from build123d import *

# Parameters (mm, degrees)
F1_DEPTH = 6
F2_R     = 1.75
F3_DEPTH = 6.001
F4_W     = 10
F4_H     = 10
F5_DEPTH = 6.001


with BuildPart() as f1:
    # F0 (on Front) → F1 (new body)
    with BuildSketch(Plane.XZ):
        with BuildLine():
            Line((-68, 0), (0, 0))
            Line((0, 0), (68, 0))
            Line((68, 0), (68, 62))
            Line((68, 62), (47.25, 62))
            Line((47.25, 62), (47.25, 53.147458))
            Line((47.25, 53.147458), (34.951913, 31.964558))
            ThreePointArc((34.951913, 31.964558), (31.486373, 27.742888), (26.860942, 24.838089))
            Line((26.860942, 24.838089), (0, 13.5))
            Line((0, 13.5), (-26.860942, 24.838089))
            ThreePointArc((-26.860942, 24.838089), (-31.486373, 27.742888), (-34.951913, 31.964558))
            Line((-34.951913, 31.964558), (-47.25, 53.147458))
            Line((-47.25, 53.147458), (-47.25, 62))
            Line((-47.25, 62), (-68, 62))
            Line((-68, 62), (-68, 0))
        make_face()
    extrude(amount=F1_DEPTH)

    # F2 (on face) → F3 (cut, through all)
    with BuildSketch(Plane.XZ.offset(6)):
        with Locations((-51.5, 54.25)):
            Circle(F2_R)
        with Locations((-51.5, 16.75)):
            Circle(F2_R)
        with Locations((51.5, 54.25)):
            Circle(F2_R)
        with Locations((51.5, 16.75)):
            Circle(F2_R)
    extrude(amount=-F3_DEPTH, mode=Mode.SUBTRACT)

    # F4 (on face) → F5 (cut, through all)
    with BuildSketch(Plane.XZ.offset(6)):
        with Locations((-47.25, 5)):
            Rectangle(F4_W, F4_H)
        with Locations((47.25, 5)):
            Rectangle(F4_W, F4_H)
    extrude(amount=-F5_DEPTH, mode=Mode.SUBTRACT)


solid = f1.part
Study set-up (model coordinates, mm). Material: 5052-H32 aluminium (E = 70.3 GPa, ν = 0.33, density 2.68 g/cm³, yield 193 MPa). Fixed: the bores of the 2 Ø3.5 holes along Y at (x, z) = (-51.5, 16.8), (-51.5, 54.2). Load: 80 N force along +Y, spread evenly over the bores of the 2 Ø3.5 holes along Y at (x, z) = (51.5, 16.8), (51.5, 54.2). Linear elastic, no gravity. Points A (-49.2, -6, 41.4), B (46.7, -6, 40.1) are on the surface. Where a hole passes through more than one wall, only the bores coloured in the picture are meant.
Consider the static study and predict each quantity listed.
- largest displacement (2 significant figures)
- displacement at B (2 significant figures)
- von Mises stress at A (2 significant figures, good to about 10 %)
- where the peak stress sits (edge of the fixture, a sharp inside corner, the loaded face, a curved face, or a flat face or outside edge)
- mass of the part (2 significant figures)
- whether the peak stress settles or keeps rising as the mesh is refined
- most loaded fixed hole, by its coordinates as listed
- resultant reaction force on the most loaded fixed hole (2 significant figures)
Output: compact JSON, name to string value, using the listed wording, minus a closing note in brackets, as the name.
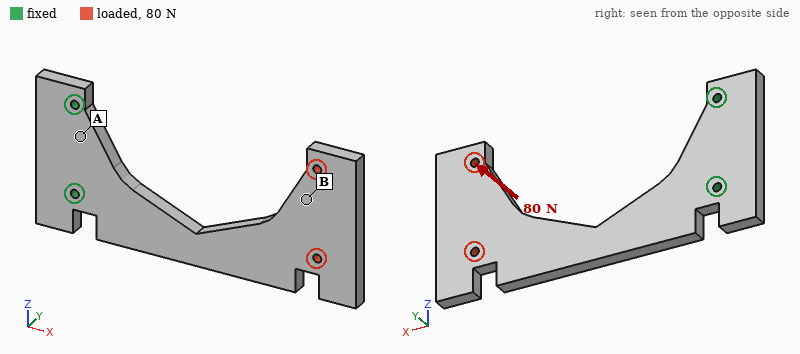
{"largest displacement": "1.7 mm", "displacement at B": "1.2 mm", "von Mises stress at A": "17 MPa", "where the peak stress sits": "edge of the fixture", "mass of the part": "78 g", "whether the peak stress settles or keeps rising as the mesh is refined": "keeps rising", "most loaded fixed hole, by its coordinates as listed": "(-51.5, 16.8)", "resultant reaction force on the most loaded fixed hole": "78 N"}
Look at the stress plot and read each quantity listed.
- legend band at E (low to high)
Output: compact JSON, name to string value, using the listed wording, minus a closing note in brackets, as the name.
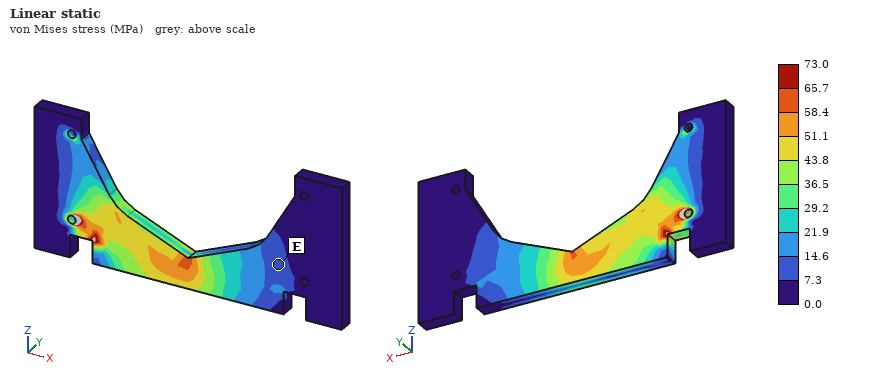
{"legend band at E": "7.3 to 14.6 MPa"}
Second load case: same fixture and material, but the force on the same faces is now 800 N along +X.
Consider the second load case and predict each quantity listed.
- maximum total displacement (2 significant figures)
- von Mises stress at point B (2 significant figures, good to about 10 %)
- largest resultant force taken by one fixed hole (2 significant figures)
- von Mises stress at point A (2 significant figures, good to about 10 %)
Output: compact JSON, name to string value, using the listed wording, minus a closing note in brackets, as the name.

{"maximum total displacement": "0.69 mm", "von Mises stress at point B": "6.7 MPa", "largest resultant force taken by one fixed hole": "430 N", "von Mises stress at point A": "6.0 MPa"}
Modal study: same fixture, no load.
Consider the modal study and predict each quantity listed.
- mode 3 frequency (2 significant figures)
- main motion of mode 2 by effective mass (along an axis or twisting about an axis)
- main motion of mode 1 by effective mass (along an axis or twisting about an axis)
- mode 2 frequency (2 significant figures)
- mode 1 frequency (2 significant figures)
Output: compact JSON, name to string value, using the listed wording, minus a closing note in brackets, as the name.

{"mode 3 frequency": "940 Hz", "main motion of mode 2 by effective mass": "along Z", "main motion of mode 1 by effective mass": "along Y", "mode 2 frequency": "710 Hz", "mode 1 frequency": "230 Hz"}
